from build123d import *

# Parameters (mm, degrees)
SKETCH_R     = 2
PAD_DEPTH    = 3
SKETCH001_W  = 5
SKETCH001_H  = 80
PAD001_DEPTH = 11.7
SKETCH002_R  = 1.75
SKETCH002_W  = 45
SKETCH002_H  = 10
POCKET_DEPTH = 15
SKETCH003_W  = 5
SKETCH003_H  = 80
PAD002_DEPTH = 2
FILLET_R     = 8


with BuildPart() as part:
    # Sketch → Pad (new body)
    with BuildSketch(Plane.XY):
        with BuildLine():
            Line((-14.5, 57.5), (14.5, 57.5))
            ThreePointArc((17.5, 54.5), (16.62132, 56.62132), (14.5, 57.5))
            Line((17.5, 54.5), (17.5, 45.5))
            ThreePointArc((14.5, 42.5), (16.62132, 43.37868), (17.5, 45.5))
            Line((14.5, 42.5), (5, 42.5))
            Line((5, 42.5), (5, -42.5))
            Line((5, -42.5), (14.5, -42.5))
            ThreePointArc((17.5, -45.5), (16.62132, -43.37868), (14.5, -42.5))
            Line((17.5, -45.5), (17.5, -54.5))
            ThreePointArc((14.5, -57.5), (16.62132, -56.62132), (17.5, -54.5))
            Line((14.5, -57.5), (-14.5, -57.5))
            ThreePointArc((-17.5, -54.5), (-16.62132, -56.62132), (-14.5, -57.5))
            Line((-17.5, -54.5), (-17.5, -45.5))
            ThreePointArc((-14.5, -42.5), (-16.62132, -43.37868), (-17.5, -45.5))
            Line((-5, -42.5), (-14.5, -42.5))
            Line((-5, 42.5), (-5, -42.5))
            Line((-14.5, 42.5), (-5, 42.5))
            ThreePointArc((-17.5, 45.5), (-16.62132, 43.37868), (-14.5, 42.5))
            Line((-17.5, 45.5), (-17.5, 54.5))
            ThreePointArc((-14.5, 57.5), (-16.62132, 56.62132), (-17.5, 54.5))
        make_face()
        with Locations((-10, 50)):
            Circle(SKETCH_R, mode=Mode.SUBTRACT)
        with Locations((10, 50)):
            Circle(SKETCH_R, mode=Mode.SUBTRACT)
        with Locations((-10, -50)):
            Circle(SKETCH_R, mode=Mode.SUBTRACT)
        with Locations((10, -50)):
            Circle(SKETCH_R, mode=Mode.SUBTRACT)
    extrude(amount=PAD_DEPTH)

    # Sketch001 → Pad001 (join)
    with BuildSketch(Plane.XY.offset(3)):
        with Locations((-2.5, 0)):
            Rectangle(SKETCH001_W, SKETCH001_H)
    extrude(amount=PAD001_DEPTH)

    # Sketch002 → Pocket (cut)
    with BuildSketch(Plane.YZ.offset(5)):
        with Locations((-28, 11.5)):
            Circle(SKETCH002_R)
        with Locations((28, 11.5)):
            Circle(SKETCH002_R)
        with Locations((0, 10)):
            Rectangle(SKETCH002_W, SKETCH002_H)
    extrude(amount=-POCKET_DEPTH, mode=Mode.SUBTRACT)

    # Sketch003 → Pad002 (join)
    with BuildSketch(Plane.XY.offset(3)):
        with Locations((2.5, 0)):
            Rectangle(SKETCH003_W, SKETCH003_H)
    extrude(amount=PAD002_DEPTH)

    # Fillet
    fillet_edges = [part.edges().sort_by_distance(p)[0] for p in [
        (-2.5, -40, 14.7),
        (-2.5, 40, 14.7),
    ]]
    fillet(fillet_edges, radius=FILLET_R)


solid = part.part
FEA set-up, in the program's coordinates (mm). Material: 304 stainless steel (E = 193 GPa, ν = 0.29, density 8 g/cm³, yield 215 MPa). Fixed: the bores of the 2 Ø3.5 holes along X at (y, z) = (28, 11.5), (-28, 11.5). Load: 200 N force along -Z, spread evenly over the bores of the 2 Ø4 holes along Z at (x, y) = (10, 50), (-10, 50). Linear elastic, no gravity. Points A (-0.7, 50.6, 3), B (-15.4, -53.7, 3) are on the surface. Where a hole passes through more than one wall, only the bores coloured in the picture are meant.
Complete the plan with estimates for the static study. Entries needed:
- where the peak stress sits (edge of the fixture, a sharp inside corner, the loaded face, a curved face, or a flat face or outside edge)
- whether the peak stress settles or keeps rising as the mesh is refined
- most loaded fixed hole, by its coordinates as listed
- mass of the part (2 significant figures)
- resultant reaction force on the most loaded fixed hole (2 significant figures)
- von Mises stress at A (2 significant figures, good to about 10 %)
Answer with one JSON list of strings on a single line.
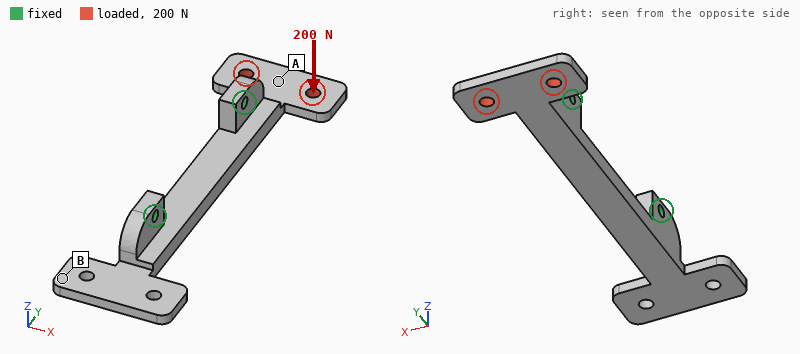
["a sharp inside corner", "keeps rising", "(28, 11.5)", "69 g", "260 N", "23 MPa"]
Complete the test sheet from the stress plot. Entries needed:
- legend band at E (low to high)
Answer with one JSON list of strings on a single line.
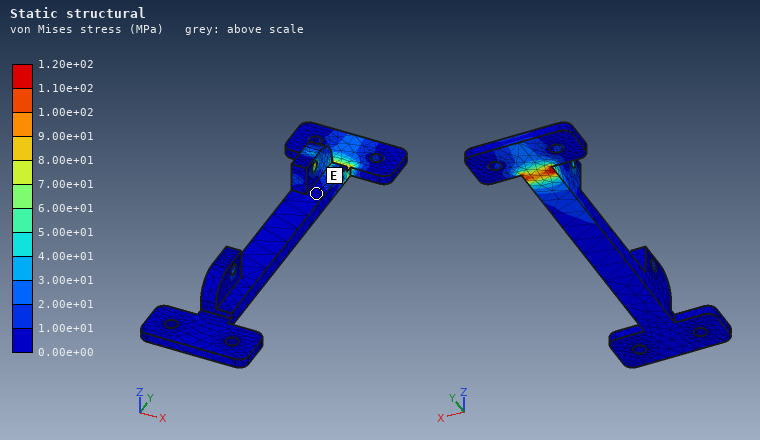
["0.00e+00 to 1.00e+01 MPa"]
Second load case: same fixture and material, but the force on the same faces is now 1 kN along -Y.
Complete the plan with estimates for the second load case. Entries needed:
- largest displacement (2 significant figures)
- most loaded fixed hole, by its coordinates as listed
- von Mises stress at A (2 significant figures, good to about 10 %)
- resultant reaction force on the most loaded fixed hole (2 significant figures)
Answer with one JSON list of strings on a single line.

["24 µm", "(28, 11.5)", "12 MPa", "610 N"]
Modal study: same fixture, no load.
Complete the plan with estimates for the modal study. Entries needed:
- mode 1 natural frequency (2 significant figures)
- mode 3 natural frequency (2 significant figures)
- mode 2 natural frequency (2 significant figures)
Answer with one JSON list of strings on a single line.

["3100 Hz", "3600 Hz", "3100 Hz"]
